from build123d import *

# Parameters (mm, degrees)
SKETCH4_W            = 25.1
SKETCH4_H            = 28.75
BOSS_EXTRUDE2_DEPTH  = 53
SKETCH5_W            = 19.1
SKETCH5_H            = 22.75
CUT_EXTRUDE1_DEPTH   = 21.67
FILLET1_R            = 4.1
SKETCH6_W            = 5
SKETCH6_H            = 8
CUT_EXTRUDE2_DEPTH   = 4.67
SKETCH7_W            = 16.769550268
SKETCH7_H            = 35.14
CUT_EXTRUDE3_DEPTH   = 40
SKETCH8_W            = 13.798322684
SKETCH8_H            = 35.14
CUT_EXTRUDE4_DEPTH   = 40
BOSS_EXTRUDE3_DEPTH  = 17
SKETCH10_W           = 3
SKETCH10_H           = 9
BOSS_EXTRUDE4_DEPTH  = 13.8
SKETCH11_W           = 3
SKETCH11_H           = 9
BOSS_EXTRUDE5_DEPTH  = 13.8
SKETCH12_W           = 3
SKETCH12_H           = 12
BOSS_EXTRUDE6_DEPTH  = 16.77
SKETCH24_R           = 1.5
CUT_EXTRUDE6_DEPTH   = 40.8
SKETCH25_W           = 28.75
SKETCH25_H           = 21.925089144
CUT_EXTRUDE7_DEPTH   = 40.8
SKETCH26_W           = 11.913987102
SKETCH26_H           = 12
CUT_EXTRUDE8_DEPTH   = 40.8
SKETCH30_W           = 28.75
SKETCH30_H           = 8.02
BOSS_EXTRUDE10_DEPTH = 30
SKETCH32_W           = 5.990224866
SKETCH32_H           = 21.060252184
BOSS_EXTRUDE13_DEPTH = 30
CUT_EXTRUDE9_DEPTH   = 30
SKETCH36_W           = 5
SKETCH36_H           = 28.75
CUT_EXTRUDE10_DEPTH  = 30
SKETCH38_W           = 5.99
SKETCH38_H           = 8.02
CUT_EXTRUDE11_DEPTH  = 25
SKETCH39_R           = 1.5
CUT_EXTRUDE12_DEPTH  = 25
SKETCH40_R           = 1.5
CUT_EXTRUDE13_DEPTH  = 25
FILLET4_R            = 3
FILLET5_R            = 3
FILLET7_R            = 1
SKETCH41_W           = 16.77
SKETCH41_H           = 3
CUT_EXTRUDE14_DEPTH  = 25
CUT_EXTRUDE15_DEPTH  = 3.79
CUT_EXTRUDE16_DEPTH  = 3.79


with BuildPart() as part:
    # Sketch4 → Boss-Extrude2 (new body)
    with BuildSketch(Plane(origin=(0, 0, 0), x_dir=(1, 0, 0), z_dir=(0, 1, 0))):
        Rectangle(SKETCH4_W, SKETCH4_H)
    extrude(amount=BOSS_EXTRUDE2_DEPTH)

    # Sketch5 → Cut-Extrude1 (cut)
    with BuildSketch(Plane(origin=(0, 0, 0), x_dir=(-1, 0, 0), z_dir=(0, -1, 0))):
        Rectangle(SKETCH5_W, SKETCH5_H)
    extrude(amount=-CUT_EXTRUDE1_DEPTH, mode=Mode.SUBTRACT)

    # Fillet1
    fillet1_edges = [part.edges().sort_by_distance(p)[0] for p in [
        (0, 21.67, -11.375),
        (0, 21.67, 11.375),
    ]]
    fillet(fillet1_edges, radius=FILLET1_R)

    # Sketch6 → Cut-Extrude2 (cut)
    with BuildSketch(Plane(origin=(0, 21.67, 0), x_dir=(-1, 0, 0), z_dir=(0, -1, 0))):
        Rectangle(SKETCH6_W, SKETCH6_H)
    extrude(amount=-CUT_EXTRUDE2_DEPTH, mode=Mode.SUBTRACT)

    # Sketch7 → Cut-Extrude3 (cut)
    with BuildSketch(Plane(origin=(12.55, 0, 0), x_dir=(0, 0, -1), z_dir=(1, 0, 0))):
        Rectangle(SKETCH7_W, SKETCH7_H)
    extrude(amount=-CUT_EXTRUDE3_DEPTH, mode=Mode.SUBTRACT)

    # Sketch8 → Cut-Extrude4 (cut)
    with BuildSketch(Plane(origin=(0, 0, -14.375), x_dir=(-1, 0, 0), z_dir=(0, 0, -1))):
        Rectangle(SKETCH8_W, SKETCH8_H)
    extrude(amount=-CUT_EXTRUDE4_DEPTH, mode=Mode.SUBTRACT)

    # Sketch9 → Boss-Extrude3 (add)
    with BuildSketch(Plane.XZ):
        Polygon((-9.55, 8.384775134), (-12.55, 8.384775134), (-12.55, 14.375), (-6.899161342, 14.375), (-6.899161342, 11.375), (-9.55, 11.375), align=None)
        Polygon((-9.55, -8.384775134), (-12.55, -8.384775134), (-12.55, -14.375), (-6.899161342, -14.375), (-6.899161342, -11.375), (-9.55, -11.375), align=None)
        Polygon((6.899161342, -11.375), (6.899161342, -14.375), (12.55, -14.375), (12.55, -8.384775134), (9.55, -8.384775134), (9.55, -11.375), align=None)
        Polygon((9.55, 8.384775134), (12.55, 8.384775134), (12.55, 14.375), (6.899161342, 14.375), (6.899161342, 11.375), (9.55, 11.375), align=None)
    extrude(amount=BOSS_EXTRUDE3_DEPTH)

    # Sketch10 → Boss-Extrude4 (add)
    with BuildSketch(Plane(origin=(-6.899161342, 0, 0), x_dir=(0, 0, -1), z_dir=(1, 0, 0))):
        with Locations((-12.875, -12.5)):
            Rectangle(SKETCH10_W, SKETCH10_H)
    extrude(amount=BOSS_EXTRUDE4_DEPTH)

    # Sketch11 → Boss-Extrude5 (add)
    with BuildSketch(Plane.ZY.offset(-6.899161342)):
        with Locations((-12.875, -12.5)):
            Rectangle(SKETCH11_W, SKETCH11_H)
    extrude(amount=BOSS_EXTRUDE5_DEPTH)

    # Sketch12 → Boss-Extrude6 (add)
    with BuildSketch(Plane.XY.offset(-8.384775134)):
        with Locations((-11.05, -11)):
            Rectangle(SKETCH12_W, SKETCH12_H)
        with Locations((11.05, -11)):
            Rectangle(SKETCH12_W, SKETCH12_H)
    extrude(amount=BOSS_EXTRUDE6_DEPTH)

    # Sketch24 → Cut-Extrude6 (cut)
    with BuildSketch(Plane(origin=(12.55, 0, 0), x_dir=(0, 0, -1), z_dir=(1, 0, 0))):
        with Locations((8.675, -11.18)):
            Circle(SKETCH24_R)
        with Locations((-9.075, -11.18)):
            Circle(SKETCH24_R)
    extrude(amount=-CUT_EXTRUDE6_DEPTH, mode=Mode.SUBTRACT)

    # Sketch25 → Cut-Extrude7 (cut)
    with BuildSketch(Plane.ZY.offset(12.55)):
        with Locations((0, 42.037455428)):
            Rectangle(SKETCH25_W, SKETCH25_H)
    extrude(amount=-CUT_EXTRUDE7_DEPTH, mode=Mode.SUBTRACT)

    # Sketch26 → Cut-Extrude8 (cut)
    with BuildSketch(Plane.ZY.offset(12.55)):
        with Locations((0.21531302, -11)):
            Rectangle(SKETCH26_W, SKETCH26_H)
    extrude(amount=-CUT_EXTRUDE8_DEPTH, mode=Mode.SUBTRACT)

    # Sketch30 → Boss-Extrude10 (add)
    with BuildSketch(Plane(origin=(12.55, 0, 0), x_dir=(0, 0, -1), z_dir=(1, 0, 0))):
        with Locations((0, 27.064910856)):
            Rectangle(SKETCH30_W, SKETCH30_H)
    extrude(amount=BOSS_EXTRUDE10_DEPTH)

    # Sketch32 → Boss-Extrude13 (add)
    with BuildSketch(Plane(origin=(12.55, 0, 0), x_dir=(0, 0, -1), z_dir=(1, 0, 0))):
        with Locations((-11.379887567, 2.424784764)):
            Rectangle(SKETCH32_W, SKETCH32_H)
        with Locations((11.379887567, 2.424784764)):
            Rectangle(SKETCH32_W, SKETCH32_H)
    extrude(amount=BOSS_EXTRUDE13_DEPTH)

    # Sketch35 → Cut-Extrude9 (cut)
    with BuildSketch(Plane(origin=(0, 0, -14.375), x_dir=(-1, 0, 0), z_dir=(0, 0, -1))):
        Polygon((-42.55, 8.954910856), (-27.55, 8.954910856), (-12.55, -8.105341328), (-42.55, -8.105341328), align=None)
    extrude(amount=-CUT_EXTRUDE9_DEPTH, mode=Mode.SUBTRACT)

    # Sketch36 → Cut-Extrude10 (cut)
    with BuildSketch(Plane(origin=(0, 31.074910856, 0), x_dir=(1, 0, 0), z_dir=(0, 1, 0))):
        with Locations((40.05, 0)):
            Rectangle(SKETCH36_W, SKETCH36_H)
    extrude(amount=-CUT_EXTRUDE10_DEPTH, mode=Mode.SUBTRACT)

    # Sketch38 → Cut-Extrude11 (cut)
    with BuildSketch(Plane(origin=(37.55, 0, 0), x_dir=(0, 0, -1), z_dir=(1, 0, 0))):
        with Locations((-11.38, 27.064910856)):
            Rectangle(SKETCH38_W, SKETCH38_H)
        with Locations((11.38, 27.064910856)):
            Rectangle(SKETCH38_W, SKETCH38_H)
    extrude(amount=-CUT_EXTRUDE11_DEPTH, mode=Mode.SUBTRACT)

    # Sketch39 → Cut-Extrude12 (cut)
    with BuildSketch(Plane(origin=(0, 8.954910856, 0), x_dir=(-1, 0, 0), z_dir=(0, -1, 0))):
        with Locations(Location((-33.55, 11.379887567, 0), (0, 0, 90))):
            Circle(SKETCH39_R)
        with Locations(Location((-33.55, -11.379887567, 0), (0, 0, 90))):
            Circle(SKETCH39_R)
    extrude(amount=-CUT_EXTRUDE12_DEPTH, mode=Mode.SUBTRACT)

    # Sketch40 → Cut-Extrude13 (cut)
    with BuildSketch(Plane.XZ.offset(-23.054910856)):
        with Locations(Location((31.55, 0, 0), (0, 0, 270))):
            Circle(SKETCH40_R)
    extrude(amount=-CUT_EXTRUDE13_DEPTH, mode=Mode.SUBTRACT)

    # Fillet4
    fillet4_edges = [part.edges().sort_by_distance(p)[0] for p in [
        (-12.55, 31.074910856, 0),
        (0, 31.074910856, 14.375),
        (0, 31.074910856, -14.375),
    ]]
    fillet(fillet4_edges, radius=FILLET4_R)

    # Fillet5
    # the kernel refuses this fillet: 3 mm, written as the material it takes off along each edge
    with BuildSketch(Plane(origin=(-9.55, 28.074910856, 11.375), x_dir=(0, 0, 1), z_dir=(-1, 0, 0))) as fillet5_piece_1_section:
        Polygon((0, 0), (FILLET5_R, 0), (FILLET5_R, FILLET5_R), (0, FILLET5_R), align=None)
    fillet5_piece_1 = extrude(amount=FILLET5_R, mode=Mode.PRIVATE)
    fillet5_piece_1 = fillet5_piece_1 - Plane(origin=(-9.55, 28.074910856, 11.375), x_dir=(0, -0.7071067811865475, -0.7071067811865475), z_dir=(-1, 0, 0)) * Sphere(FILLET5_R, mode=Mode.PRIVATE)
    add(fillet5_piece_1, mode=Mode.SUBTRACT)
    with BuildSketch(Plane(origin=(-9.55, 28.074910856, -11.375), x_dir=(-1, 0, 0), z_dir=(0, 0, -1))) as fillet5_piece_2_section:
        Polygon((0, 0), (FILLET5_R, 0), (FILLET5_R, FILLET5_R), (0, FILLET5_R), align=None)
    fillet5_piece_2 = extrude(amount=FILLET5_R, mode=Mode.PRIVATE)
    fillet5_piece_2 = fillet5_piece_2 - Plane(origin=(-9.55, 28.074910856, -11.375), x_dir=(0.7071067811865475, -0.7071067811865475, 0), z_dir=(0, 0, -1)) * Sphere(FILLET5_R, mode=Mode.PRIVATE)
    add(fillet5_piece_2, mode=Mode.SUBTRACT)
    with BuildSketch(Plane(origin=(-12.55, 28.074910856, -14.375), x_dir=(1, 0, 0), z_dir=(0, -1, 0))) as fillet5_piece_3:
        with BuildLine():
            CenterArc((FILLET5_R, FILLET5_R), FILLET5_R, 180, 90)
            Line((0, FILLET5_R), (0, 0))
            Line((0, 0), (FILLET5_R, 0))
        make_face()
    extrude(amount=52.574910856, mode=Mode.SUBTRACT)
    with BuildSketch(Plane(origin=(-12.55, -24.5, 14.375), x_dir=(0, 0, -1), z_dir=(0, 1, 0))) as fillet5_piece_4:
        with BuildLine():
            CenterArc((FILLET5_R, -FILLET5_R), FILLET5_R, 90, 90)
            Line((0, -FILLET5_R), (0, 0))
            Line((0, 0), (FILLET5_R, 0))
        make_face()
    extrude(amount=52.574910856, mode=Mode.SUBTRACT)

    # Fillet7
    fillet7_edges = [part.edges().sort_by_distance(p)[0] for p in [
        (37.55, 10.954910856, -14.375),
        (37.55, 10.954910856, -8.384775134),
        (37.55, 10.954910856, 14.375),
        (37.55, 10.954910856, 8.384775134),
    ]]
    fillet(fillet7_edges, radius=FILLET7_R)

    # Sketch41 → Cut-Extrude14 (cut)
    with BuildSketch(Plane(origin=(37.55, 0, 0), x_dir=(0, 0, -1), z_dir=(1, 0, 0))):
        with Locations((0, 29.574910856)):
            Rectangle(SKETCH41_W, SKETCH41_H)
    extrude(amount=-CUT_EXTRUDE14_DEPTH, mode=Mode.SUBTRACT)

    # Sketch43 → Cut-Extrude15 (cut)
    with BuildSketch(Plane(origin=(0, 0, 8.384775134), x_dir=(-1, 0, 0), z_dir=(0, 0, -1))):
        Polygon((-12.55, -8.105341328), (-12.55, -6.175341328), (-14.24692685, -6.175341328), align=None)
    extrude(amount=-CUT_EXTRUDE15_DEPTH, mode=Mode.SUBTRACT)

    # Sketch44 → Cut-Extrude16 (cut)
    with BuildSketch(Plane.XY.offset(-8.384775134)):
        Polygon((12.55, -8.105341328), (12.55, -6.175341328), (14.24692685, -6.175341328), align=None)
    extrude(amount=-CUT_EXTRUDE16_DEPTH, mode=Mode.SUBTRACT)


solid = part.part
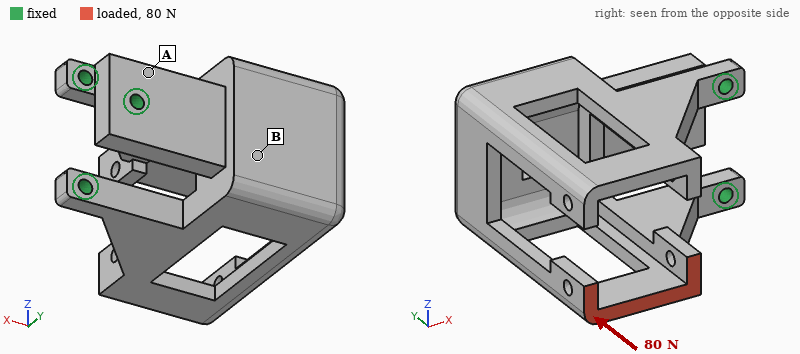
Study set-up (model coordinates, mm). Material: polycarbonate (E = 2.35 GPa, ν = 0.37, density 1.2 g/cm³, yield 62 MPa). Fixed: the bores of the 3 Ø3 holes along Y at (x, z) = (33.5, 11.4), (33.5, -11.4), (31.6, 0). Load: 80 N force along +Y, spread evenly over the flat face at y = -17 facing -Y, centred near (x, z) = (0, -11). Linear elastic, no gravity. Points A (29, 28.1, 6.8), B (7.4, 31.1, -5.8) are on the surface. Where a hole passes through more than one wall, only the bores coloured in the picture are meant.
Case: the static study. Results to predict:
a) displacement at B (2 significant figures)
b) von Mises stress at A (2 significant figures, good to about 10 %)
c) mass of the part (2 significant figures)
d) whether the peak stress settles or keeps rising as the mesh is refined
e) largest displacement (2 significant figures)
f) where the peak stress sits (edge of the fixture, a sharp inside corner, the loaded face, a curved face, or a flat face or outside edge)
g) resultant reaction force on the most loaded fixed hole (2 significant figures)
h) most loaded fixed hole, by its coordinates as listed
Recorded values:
0.26 mm
3.7 MPa
20 g
keeps rising
0.76 mm
edge of the fixture
120 N
(31.6, 0)
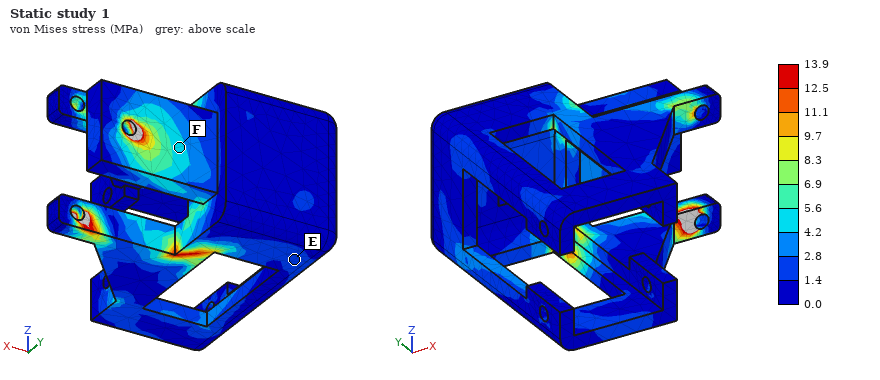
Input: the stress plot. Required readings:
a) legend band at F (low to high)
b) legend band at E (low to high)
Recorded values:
4.2 to 5.6 MPa
1.4 to 2.8 MPa
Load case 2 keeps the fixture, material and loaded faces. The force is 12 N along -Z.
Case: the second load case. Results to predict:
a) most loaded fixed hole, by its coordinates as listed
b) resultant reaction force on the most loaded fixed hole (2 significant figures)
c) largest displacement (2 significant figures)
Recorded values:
(33.5, -11.4)
8.0 N
0.85 mm
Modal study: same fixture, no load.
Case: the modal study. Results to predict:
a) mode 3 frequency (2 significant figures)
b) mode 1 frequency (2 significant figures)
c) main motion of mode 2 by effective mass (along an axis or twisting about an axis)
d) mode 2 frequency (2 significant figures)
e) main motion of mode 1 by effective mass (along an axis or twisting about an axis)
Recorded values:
750 Hz
440 Hz
along Y
680 Hz
along Z
